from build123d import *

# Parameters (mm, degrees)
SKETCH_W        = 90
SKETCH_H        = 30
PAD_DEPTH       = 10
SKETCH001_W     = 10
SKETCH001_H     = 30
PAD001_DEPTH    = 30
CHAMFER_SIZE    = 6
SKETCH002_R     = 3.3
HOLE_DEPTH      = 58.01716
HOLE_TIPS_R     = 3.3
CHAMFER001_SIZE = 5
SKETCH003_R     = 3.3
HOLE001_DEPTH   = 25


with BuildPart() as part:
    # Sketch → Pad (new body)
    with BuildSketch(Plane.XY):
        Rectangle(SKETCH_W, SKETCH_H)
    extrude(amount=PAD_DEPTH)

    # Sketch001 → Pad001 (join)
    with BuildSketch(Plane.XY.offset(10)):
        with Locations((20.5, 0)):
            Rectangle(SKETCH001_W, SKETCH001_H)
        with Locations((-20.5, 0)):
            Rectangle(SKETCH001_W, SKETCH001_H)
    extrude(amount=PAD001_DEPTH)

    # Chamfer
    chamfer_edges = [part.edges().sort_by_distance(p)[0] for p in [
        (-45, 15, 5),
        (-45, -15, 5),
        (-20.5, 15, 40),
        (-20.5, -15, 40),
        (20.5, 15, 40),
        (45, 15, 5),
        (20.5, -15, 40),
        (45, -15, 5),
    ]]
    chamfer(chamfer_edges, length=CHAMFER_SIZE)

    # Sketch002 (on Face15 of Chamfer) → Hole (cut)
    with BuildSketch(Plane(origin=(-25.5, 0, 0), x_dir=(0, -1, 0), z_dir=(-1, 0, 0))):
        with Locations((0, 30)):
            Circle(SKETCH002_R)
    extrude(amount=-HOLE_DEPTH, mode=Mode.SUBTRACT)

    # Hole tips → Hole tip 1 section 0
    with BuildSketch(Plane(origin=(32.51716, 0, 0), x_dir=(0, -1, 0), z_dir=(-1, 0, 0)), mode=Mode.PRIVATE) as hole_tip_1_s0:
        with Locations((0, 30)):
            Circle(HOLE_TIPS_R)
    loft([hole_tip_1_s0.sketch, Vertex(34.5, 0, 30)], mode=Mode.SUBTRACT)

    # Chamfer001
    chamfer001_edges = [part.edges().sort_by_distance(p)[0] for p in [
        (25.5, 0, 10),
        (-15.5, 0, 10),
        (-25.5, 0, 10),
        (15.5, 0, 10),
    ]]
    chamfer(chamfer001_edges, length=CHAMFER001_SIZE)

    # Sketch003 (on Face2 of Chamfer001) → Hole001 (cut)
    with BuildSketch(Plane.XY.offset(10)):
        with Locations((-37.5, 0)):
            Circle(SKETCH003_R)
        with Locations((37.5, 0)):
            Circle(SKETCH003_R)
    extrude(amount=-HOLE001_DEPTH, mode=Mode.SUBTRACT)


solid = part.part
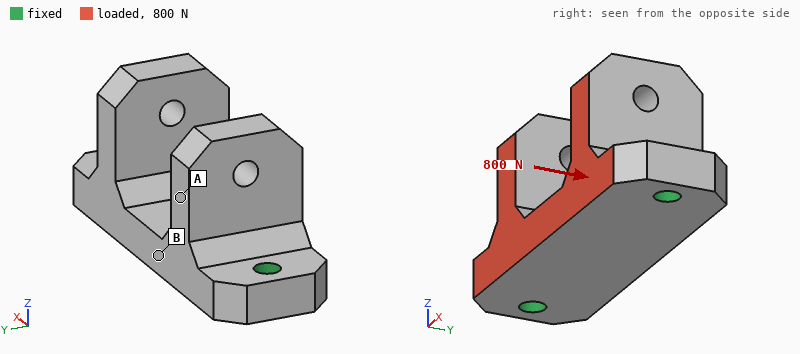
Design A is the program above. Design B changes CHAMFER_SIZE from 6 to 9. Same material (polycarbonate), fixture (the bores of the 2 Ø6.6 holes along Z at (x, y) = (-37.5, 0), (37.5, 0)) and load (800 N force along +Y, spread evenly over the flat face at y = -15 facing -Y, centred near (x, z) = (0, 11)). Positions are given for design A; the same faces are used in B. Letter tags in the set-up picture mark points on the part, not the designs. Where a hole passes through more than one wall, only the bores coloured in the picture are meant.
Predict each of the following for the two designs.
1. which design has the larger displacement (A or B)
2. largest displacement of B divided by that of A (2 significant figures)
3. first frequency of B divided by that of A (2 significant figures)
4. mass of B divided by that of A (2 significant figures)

A
0.92
1.0
0.96
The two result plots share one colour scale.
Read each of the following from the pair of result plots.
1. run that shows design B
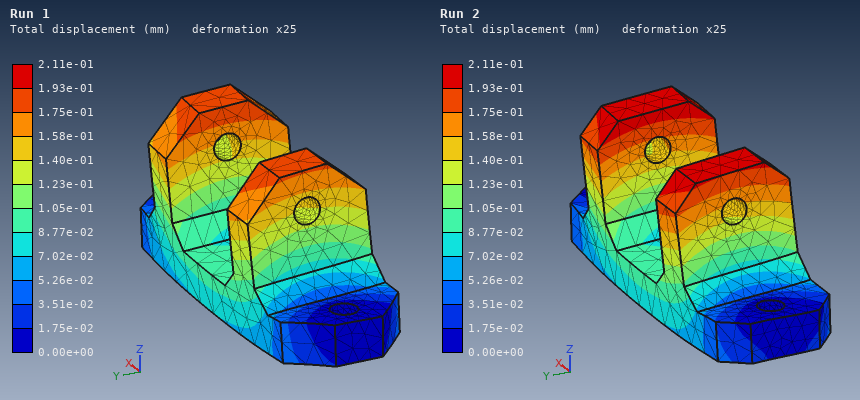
Run 1
